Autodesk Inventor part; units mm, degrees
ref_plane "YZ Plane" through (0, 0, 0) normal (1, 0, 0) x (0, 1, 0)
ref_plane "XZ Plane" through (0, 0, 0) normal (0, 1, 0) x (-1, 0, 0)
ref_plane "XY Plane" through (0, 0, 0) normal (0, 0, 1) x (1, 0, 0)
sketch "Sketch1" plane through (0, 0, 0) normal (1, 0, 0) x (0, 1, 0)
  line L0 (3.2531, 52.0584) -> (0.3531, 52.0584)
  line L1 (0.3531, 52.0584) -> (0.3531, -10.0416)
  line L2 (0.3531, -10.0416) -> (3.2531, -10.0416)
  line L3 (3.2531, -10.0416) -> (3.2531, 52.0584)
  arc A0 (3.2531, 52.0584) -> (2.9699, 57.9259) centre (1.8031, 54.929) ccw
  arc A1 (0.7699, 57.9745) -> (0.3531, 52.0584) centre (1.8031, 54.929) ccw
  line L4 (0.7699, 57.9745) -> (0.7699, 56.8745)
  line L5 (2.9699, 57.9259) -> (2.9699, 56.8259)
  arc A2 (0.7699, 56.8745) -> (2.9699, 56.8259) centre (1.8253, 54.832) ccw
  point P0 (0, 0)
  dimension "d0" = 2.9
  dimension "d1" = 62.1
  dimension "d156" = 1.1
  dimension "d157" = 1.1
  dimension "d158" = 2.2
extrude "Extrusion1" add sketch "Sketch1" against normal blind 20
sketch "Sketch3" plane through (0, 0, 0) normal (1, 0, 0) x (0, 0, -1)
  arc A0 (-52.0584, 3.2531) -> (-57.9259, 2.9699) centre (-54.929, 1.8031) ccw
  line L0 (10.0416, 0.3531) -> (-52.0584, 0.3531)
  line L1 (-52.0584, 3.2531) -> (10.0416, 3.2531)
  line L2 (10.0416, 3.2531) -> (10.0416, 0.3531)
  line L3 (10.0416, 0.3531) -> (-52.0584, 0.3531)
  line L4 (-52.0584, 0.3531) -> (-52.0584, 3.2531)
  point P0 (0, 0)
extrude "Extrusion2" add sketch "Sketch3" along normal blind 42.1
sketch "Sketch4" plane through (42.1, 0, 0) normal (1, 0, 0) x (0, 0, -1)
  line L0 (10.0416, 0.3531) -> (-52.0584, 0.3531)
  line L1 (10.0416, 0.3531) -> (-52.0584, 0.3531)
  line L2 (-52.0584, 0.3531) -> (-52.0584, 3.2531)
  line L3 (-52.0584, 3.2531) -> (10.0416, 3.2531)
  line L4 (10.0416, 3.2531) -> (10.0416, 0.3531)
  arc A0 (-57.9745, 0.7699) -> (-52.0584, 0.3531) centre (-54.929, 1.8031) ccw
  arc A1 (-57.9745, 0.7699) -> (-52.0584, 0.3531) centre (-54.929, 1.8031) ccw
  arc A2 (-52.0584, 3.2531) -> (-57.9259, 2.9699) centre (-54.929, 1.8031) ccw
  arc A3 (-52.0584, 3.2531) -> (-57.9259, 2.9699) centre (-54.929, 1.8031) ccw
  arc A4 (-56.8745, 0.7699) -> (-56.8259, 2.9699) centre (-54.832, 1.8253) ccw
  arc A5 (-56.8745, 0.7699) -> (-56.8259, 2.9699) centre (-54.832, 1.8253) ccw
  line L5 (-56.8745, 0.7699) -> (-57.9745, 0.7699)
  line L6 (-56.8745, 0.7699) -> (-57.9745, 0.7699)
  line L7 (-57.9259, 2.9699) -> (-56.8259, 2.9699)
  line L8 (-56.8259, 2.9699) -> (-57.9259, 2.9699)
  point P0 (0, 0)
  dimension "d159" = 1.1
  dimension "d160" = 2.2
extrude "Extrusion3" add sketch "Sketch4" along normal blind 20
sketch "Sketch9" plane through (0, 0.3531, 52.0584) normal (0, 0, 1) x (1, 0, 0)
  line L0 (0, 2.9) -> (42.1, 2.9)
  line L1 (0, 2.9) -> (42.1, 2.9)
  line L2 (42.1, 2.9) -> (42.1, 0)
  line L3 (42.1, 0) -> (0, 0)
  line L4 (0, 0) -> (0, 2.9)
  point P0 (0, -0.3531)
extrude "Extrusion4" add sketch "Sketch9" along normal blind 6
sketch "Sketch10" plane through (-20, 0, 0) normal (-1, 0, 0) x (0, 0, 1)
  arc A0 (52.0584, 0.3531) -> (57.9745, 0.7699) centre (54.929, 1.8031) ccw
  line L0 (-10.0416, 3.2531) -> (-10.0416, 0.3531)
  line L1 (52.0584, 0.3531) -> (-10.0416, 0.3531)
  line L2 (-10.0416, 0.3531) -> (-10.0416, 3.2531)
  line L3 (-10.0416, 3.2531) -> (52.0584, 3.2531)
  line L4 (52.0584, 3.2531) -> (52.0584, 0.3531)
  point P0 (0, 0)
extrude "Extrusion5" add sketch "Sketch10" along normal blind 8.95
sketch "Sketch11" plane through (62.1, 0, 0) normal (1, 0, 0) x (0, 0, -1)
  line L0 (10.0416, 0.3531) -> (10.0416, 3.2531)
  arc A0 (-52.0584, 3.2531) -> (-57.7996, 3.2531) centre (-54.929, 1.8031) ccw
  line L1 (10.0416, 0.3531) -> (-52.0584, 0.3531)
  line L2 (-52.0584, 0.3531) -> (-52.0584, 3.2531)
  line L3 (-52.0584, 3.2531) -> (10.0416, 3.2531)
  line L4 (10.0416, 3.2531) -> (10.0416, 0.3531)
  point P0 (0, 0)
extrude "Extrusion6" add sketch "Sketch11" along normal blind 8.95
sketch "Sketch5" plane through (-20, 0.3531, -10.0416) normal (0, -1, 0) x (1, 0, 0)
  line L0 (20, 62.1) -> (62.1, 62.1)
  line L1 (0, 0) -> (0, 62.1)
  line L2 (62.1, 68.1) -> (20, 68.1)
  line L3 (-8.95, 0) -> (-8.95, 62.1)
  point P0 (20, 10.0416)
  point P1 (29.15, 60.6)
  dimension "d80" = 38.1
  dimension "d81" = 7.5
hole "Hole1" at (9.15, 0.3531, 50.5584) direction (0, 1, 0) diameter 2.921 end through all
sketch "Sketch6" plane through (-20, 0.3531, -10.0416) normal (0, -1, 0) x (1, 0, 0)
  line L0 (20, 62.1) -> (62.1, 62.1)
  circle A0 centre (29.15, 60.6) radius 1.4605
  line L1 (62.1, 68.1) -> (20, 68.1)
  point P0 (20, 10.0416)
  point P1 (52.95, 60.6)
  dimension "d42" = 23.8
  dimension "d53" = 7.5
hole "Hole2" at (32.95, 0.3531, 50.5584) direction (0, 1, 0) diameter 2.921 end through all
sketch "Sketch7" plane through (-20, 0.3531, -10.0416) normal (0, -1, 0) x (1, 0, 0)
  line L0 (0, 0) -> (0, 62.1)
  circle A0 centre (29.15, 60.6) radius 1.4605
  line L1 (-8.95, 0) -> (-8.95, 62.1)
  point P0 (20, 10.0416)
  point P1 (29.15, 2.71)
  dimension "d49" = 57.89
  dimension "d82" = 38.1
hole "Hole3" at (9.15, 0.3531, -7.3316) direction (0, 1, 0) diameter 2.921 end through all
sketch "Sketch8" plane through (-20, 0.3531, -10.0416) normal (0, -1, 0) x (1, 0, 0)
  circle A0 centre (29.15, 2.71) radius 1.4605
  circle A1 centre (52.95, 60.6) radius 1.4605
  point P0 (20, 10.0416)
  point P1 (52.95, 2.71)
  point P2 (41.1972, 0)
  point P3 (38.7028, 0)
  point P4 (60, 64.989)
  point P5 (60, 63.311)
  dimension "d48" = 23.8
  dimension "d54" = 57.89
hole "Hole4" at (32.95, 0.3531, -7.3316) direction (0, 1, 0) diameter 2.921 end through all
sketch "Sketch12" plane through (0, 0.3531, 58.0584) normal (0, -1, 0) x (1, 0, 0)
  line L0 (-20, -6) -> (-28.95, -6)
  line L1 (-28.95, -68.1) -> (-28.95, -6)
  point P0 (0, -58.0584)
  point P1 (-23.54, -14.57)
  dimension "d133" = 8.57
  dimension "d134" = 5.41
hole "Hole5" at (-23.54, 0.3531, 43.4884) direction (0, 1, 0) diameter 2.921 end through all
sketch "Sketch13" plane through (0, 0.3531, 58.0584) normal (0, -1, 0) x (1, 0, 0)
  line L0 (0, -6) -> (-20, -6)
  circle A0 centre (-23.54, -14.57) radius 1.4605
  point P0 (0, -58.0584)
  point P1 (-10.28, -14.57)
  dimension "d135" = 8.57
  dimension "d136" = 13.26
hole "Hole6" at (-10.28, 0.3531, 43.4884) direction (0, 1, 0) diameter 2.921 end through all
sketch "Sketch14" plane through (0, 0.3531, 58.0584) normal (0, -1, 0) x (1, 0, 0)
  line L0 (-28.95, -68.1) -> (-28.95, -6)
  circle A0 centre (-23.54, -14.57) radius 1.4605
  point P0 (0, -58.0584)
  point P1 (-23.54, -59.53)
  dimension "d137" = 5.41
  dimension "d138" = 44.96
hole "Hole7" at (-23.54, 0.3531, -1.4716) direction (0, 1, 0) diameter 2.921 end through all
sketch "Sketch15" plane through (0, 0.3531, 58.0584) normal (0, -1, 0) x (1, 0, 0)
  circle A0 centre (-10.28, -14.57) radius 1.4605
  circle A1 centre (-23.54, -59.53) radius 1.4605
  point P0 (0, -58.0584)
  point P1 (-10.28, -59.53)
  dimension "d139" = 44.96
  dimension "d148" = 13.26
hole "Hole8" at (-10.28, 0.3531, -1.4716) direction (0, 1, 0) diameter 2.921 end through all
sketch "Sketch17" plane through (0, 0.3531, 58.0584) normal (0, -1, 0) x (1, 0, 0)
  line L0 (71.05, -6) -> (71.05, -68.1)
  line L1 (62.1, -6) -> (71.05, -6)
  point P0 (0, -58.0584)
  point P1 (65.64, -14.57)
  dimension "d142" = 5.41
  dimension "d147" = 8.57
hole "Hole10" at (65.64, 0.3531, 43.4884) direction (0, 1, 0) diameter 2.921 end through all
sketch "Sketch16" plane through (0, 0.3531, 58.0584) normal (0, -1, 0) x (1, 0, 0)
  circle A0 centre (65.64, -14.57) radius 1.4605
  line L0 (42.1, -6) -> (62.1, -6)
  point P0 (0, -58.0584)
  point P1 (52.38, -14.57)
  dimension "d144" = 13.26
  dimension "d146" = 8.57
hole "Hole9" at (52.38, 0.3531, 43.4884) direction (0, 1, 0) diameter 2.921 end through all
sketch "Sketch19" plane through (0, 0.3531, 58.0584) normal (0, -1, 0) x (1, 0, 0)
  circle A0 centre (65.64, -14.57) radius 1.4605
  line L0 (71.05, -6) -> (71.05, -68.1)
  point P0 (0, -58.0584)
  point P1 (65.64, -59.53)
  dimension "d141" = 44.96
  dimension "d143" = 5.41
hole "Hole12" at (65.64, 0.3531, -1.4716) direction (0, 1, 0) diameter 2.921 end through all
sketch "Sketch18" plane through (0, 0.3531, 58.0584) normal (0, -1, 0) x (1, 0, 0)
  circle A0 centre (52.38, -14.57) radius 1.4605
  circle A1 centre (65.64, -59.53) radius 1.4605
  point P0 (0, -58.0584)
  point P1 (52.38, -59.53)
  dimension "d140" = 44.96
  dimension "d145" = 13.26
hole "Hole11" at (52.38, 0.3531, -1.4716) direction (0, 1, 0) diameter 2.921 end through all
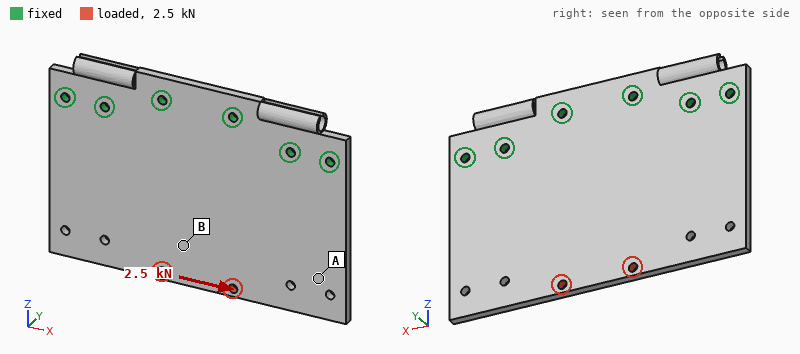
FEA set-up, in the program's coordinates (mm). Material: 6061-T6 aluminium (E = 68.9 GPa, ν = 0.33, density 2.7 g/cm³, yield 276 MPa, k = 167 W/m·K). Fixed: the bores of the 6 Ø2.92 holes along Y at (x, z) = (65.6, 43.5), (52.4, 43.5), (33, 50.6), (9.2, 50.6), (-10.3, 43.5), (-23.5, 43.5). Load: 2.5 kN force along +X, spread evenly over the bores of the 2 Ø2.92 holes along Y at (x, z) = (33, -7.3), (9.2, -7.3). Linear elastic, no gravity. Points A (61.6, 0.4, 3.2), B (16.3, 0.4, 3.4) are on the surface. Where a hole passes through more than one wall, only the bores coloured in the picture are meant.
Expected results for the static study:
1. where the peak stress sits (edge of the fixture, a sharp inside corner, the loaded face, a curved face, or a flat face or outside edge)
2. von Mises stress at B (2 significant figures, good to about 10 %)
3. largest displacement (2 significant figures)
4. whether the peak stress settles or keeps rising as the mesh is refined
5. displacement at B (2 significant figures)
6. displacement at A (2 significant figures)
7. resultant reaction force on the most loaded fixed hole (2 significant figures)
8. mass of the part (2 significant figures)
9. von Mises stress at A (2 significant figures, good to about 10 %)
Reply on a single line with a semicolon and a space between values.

edge of the fixture; 24 MPa; 33 µm; keeps rising; 22 µm; 22 µm; 1.1 kN; 51 g; 7.2 MPa
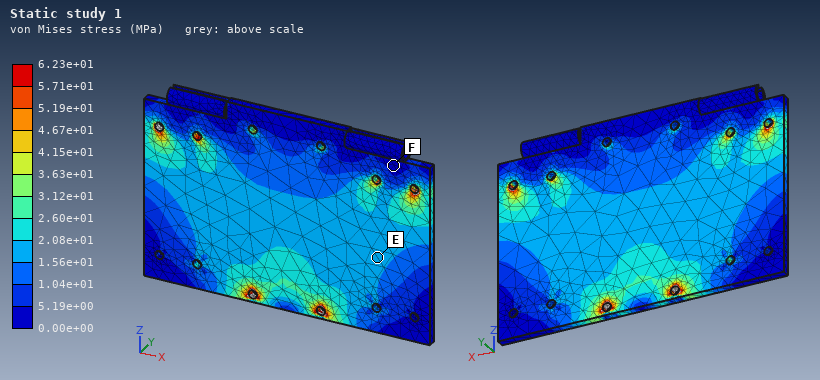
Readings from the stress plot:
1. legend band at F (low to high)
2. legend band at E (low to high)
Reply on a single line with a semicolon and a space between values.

0.00e+00 to 5.19e+00 MPa; 1.56e+01 to 2.08e+01 MPa
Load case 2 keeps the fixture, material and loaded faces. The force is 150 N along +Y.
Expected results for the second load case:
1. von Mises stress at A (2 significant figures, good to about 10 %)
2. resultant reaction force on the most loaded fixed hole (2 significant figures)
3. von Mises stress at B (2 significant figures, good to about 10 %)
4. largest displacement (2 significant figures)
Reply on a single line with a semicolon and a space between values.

14 MPa; 130 N; 22 MPa; 0.64 mm
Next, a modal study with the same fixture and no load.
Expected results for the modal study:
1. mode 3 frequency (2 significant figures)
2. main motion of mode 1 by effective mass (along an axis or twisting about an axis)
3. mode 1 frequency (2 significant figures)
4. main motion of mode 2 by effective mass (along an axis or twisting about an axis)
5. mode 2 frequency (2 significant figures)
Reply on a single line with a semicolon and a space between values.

2600 Hz; along Y; 780 Hz; twisting about Z; 1300 Hz
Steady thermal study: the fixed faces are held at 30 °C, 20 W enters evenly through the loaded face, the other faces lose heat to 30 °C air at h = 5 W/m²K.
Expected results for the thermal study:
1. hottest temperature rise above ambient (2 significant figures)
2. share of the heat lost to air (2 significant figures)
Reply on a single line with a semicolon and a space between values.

35 K; 3.6 %
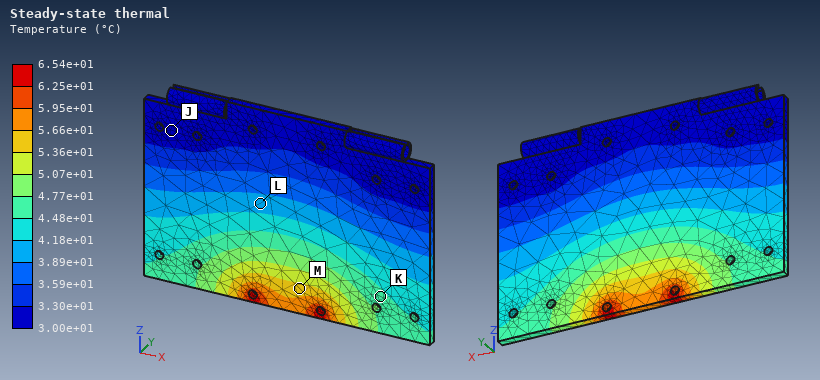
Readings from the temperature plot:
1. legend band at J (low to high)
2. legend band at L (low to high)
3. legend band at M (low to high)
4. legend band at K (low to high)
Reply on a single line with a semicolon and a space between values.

3.00e+01 to 3.30e+01 °C; 3.89e+01 to 4.18e+01 °C; 5.36e+01 to 5.66e+01 °C; 4.48e+01 to 4.77e+01 °C
